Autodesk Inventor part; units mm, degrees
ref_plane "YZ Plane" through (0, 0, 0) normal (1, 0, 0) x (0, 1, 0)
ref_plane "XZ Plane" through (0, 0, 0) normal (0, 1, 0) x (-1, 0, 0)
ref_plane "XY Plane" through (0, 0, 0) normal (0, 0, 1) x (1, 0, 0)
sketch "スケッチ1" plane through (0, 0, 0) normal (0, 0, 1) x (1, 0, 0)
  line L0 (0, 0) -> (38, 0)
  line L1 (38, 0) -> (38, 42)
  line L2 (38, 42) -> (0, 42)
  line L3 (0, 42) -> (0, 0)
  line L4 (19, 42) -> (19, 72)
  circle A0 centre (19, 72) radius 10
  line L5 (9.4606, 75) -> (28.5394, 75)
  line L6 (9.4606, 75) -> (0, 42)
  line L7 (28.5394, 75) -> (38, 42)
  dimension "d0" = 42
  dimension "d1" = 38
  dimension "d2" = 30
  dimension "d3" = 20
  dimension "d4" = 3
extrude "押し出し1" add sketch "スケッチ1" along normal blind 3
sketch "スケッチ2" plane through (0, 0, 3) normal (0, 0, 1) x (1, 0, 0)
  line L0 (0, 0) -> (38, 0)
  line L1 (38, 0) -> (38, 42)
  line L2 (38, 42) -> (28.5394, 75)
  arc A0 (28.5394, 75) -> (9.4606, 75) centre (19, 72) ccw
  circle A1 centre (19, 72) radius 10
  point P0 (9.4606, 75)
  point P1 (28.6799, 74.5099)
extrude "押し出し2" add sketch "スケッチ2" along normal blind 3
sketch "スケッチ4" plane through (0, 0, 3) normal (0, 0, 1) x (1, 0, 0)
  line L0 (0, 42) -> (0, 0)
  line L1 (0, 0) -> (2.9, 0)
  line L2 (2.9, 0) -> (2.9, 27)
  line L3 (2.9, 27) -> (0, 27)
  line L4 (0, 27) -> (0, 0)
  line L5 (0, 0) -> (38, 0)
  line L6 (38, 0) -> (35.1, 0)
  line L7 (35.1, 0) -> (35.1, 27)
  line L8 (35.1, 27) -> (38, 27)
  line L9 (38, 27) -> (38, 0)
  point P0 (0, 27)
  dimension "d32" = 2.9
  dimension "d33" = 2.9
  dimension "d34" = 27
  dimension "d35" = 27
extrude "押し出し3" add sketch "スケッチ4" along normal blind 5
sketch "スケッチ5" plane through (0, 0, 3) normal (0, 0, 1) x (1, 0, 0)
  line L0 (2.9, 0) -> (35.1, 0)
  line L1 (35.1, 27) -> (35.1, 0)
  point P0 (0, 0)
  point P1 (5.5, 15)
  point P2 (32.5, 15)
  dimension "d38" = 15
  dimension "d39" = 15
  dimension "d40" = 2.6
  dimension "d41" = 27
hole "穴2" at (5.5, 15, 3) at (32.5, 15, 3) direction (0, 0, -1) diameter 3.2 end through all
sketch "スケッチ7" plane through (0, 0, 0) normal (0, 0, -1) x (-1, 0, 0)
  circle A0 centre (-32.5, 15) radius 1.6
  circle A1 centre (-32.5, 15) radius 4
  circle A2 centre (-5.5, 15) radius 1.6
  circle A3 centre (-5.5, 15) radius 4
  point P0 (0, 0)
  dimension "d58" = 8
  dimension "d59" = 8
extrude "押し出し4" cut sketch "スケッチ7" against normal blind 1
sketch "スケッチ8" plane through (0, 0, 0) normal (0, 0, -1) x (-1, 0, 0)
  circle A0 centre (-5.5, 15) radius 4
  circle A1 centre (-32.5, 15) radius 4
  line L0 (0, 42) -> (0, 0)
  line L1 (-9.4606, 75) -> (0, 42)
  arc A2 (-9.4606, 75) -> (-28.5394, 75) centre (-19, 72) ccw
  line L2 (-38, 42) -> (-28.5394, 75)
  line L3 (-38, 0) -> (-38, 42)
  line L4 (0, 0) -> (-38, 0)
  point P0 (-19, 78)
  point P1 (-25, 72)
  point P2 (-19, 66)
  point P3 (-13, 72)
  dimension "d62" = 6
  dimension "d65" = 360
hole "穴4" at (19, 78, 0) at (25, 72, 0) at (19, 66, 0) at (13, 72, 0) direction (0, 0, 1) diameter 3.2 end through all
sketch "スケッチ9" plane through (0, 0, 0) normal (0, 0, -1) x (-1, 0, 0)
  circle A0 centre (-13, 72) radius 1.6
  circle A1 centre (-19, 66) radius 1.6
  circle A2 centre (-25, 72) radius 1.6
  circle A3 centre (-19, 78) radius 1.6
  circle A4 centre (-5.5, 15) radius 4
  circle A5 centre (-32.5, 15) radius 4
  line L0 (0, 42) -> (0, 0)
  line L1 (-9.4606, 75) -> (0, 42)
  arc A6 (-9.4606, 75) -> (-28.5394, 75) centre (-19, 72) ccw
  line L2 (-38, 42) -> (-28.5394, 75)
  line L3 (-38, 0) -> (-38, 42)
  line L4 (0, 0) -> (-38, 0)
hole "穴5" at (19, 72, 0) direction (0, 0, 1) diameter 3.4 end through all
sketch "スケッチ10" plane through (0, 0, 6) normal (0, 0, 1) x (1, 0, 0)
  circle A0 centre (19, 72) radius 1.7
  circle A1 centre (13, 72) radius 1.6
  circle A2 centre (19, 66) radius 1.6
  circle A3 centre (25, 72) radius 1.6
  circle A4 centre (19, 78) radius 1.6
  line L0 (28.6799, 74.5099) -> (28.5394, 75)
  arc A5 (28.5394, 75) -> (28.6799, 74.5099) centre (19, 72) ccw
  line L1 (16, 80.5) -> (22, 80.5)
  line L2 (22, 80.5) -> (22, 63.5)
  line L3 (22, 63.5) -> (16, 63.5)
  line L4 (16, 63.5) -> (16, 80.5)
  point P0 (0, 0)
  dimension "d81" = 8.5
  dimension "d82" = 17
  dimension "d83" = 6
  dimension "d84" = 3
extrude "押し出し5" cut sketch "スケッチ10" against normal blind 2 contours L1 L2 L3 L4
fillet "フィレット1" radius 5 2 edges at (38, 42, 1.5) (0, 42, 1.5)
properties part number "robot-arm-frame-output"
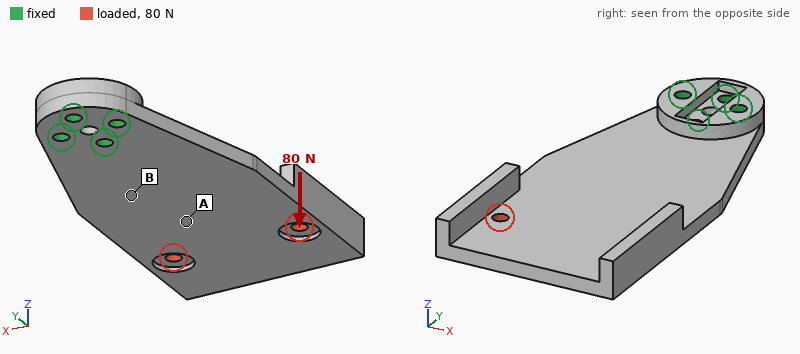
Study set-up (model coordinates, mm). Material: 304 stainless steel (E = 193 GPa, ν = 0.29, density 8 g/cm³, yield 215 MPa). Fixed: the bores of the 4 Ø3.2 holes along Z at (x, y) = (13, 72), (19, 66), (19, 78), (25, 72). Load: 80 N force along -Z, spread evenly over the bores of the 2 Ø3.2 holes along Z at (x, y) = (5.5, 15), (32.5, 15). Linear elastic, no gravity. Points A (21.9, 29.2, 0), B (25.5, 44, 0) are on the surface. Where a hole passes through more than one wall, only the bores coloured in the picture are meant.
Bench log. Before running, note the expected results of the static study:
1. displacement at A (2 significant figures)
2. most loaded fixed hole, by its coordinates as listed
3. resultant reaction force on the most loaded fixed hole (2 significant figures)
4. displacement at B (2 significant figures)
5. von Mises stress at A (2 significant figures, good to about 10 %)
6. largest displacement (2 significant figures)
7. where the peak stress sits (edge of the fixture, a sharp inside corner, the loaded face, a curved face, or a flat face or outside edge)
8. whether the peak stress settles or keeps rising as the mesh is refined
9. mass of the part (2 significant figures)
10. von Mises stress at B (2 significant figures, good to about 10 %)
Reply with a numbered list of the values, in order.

1. 0.15 mm
2. (19, 66)
3. 340 N
4. 0.061 mm
5. 17 MPa
6. 0.35 mm
7. edge of the fixture
8. keeps rising
9. 73 g
10. 40 MPa
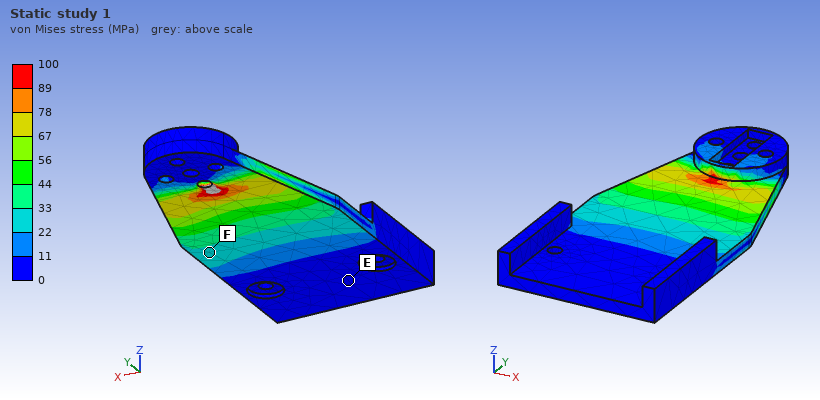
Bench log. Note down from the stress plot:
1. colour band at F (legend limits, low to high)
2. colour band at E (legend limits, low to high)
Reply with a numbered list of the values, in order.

1. 22 to 33 MPa
2. 0 to 11 MPa
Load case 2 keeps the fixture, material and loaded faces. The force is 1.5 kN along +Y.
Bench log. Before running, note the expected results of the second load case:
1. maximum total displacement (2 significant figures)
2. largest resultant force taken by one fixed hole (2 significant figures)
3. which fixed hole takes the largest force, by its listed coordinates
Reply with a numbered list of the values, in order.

1. 91 µm
2. 630 N
3. (19, 66)
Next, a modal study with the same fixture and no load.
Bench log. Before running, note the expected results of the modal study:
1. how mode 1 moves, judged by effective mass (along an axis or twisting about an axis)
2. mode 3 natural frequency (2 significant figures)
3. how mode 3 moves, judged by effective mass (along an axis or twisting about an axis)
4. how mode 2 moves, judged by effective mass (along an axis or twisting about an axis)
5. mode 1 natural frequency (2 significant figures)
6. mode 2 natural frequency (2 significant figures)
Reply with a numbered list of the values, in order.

1. along Z
2. 2900 Hz
3. along X
4. twisting about Y
5. 470 Hz
6. 1500 Hz
